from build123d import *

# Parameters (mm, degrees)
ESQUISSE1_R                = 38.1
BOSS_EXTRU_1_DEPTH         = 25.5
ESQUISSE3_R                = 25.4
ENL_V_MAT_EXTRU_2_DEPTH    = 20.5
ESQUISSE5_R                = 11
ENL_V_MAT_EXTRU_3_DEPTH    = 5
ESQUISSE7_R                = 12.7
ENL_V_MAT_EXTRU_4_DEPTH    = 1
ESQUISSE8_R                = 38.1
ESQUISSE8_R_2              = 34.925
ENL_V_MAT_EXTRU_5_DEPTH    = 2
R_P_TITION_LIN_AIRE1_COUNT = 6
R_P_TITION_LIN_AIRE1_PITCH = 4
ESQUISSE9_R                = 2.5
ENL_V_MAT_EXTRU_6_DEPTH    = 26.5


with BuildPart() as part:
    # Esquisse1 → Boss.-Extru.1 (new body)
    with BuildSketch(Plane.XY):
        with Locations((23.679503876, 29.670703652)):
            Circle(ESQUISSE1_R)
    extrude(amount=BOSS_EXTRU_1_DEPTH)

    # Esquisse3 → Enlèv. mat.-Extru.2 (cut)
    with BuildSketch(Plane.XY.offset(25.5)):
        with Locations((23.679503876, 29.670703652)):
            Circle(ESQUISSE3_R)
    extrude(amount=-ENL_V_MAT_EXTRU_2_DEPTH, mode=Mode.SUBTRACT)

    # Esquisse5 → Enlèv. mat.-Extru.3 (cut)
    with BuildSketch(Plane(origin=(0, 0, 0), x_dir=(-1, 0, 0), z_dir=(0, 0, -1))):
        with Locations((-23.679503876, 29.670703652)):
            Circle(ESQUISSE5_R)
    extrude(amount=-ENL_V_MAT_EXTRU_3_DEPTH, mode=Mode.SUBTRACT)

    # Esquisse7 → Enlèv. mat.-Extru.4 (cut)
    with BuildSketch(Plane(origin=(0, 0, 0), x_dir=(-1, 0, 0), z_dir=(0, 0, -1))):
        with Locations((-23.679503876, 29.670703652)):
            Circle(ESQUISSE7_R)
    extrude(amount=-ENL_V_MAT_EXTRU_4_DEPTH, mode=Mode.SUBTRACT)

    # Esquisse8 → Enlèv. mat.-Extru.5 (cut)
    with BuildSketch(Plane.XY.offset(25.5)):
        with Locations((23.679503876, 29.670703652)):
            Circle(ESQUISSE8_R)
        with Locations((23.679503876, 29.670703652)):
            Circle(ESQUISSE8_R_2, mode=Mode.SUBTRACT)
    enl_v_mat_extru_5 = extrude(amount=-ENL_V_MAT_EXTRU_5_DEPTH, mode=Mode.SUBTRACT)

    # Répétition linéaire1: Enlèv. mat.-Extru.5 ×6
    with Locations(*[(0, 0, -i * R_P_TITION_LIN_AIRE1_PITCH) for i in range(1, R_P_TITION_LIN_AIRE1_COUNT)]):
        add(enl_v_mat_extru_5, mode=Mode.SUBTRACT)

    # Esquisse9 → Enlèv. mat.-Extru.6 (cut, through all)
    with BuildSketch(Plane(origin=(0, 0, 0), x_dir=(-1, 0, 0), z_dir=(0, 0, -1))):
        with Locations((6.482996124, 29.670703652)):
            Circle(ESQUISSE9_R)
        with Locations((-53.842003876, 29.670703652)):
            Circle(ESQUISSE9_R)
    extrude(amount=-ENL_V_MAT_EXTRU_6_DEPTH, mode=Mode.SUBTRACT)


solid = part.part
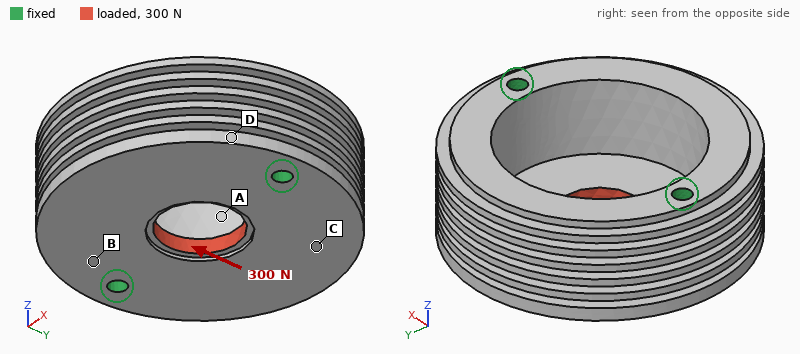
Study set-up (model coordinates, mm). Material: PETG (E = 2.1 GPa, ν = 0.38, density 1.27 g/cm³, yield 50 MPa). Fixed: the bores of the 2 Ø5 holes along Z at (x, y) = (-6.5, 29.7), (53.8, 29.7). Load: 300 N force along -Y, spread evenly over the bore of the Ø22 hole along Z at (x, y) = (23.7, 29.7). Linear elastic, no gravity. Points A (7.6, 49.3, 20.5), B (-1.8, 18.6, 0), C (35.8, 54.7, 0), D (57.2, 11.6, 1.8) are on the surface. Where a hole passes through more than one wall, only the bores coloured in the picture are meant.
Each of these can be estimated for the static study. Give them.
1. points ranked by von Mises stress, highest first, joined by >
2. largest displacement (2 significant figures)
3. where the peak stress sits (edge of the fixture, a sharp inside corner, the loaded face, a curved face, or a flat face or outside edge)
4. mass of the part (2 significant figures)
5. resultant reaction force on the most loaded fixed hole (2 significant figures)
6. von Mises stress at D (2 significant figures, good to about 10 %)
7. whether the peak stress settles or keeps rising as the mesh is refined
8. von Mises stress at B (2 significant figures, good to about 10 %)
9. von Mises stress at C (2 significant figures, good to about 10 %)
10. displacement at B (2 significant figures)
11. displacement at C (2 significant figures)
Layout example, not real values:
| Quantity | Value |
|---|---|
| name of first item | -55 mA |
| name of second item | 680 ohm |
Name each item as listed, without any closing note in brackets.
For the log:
| Quantity | Value |
|---|---|
| points ranked by von Mises stress, highest first, joined by > | B > C > D > A |
| largest displacement | 21 µm |
| where the peak stress sits | edge of the fixture |
| mass of the part | 80 g |
| resultant reaction force on the most loaded fixed hole | 150 N |
| von Mises stress at D | 0.35 MPa |
| whether the peak stress settles or keeps rising as the mesh is refined | keeps rising |
| von Mises stress at B | 0.79 MPa |
| von Mises stress at C | 0.61 MPa |
| displacement at B | 6.3 µm |
| displacement at C | 15 µm |
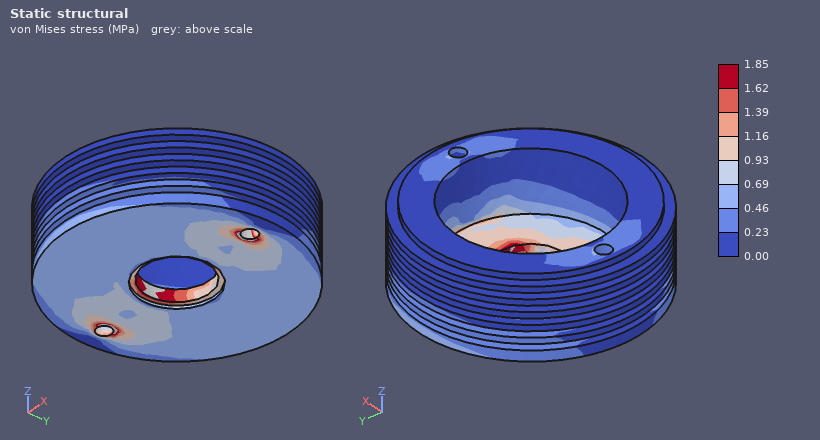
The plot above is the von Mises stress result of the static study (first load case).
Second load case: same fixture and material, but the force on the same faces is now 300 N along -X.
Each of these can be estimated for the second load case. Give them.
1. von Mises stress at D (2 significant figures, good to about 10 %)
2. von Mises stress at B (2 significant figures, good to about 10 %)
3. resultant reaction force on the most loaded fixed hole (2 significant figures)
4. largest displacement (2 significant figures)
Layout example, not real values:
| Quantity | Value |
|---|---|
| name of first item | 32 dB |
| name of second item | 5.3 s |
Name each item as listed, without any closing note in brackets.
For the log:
| Quantity | Value |
|---|---|
| von Mises stress at D | 0.27 MPa |
| von Mises stress at B | 0.46 MPa |
| resultant reaction force on the most loaded fixed hole | 150 N |
| largest displacement | 16 µm |
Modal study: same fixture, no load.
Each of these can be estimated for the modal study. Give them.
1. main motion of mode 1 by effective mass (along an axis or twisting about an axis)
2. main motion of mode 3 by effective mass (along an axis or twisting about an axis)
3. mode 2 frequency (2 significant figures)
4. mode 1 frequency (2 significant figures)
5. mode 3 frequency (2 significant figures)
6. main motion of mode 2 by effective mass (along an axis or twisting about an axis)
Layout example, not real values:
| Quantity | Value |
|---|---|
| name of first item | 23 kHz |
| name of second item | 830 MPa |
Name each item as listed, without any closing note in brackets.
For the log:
| Quantity | Value |
|---|---|
| main motion of mode 1 by effective mass | twisting about X |
| main motion of mode 3 by effective mass | twisting about Z |
| mode 2 frequency | 2300 Hz |
| mode 1 frequency | 2100 Hz |
| mode 3 frequency | 2900 Hz |
| main motion of mode 2 by effective mass | along Z |
